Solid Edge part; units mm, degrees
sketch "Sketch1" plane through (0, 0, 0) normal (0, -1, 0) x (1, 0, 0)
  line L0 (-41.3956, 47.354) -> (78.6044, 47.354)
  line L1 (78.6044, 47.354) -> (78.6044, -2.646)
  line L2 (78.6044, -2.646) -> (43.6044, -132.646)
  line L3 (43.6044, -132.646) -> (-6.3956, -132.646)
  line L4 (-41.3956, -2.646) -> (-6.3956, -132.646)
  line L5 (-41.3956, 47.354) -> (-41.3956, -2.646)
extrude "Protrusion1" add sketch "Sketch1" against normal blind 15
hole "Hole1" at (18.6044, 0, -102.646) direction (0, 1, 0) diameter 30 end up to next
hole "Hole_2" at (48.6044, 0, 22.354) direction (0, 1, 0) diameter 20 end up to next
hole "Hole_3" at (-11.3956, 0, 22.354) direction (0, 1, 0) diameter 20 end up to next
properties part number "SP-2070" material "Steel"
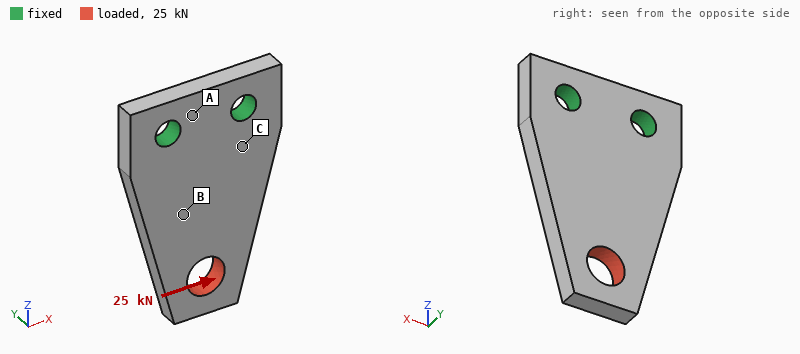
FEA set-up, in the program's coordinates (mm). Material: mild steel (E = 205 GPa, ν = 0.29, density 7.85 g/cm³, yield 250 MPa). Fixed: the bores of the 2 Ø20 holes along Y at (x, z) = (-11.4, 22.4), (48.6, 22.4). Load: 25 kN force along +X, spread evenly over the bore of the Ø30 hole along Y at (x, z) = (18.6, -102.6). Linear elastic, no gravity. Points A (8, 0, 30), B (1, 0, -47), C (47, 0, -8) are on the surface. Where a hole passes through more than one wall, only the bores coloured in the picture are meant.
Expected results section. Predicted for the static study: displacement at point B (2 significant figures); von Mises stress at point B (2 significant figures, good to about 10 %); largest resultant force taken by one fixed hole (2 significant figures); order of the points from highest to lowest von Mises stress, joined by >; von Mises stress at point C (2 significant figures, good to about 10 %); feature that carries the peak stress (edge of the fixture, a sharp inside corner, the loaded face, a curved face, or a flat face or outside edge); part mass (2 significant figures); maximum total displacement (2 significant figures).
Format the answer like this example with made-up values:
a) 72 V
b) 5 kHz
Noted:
a) 0.033 mm
b) 36 MPa
c) 43 kN
d) C > B > A
e) 58 MPa
f) edge of the fixture
g) 1.9 kg
h) 0.12 mm
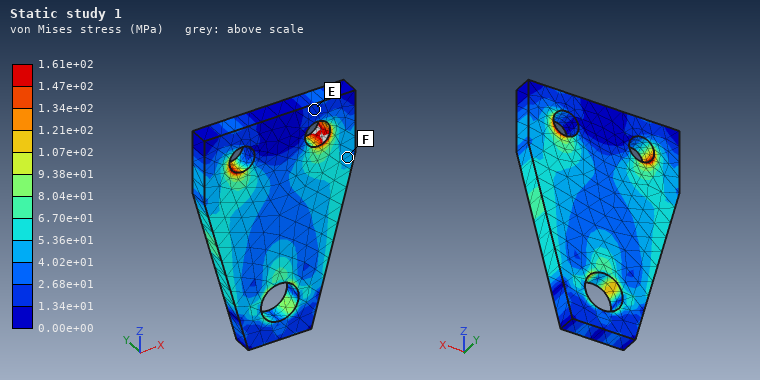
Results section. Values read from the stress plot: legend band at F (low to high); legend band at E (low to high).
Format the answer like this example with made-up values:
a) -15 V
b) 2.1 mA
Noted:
a) 4.02e+01 to 5.36e+01 MPa
b) 1.34e+01 to 2.68e+01 MPa
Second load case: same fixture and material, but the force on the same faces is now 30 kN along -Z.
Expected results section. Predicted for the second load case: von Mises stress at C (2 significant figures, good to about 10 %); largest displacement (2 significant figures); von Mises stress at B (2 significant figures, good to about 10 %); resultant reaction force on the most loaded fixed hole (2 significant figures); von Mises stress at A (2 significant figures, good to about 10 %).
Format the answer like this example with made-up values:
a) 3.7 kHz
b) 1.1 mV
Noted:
a) 22 MPa
b) 22 µm
c) 22 MPa
d) 15 kN
e) 7.8 MPa
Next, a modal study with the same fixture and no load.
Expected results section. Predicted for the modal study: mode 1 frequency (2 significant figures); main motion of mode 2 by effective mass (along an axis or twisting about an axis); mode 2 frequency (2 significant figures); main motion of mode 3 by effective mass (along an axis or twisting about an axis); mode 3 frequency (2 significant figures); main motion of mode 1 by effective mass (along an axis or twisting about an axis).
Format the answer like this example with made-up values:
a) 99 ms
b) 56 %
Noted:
a) 770 Hz
b) twisting about Z
c) 2700 Hz
d) along Y
e) 3400 Hz
f) along Y
